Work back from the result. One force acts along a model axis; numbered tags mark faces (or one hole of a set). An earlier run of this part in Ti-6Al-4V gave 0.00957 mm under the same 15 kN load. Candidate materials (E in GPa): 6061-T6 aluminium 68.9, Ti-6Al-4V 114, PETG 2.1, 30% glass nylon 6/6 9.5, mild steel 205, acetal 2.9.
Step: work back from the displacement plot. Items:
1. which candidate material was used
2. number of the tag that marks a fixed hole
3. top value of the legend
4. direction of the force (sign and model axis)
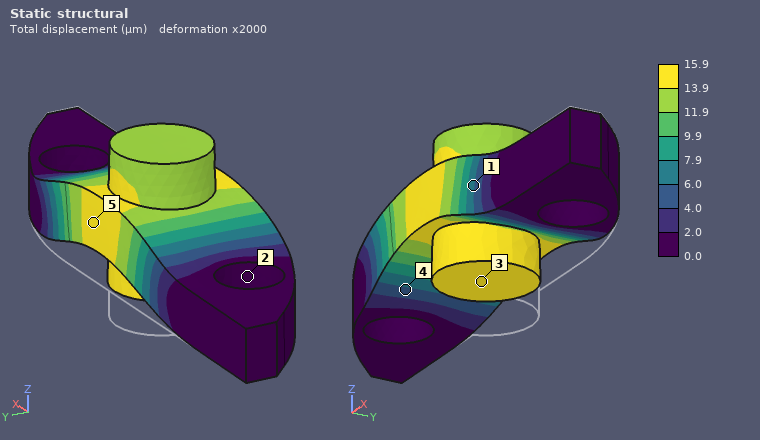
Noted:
6061-T6 aluminium
2
15.9 µm
+Z
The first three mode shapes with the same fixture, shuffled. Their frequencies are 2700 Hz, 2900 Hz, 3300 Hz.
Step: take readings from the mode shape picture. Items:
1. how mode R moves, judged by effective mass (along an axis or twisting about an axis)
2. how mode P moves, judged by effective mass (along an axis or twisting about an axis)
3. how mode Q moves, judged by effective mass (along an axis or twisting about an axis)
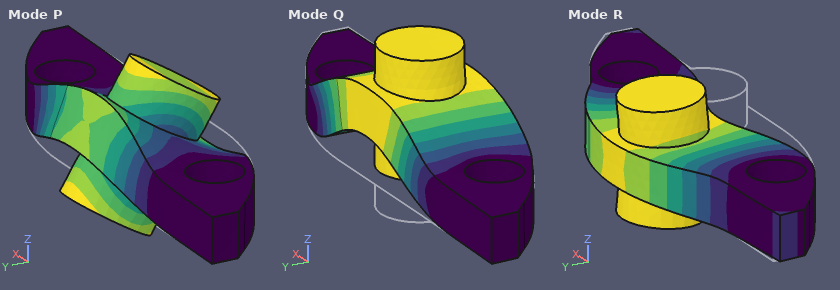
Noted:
along Y
twisting about X
along Z
